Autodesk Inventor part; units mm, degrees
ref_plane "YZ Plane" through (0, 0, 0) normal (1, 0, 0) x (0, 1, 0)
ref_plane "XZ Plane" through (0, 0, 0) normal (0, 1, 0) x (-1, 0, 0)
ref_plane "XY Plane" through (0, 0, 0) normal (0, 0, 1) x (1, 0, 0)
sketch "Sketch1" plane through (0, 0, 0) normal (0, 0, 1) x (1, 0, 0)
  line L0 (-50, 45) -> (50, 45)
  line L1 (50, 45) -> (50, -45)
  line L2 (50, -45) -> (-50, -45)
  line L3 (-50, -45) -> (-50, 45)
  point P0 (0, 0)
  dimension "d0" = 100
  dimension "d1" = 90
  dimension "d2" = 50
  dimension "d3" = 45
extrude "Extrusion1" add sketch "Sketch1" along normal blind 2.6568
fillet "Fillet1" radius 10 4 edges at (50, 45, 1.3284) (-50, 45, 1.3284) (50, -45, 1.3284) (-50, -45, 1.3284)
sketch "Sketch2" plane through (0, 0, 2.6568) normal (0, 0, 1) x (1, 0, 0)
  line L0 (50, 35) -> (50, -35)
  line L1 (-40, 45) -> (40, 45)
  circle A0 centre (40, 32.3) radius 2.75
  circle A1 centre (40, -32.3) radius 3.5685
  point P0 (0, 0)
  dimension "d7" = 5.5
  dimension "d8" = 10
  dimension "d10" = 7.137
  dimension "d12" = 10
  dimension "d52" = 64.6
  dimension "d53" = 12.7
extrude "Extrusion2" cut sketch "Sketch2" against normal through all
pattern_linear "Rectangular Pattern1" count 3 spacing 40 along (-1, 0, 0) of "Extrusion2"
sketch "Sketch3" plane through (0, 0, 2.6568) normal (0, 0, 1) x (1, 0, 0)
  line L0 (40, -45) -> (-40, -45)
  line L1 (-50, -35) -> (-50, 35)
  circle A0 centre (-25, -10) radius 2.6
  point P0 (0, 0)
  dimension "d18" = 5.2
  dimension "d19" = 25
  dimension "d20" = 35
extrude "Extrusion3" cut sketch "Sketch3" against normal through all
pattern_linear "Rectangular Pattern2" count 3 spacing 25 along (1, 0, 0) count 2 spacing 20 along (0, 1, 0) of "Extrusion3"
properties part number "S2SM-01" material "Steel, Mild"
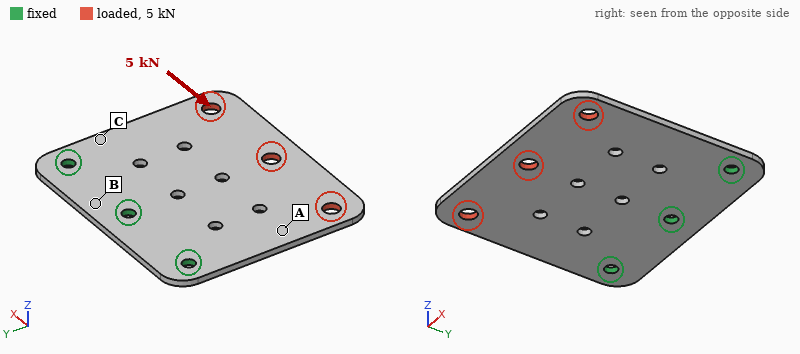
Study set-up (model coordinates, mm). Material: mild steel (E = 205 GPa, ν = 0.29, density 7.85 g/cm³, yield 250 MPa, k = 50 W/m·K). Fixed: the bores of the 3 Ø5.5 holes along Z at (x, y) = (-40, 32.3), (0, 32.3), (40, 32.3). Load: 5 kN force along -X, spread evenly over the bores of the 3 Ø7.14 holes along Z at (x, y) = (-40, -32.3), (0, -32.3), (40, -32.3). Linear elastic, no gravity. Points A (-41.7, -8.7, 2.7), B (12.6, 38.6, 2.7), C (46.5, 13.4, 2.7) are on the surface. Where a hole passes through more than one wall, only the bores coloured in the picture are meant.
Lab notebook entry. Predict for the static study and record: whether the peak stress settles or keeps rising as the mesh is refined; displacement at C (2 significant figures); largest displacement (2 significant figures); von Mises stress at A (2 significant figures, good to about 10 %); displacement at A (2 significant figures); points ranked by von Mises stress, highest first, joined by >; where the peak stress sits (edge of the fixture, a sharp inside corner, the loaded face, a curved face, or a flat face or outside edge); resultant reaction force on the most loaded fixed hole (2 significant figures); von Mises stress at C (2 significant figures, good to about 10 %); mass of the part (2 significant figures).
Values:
keeps rising
12 µm
39 µm
30 MPa
22 µm
C > A > B
edge of the fixture
4.2 kN
55 MPa
180 g
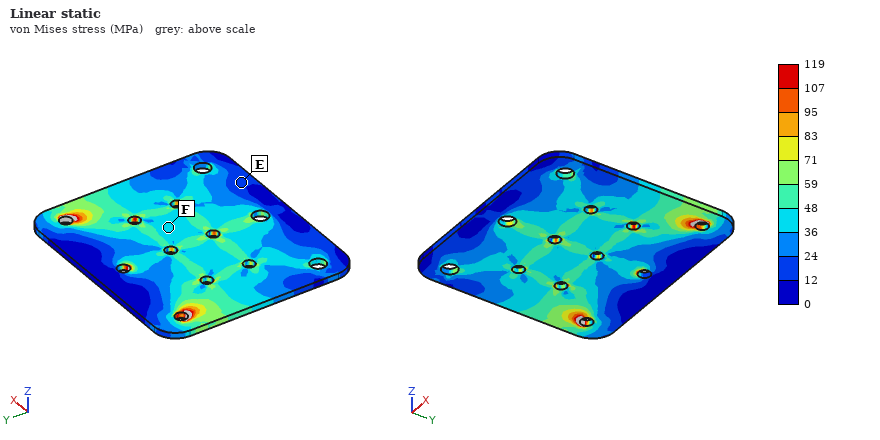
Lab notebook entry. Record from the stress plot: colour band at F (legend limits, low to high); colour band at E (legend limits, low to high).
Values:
36 to 48 MPa
12 to 24 MPa
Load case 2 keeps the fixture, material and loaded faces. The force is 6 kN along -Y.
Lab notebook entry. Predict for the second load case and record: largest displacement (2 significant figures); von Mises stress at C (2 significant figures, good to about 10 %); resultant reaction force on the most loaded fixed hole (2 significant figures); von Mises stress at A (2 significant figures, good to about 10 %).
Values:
11 µm
28 MPa
2.1 kN
28 MPa
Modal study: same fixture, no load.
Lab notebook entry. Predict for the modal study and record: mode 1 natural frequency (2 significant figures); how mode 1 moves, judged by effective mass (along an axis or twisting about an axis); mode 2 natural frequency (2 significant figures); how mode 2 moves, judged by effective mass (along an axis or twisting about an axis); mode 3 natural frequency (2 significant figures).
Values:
380 Hz
along Z
790 Hz
twisting about Y
1900 Hz
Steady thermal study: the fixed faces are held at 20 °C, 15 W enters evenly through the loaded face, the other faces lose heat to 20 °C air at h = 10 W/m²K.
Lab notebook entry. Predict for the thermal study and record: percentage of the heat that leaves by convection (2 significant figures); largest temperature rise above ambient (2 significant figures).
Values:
36 %
68 K
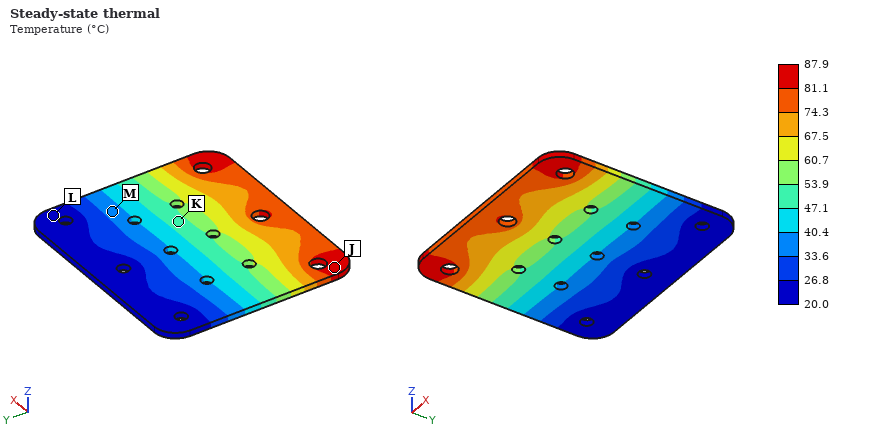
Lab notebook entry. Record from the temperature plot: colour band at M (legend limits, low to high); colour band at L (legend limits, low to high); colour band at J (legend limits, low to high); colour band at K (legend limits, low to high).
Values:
33.6 to 40.4 °C
20.0 to 26.8 °C
81.1 to 87.9 °C
47.1 to 53.9 °C
